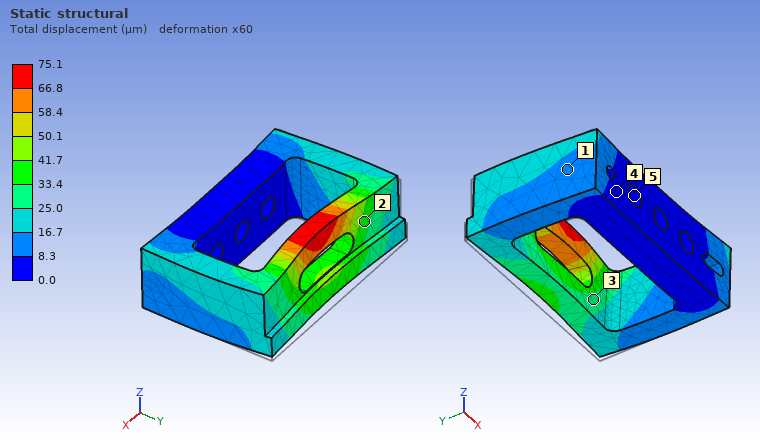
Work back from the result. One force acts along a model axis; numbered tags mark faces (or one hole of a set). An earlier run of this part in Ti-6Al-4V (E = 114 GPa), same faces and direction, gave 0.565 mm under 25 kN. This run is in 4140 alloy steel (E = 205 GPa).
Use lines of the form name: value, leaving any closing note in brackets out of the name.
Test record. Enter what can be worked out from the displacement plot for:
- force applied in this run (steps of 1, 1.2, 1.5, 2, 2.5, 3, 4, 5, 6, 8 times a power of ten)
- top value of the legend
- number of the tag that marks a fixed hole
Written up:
force applied in this run: 6 kN
top value of the legend: 75.1 µm
number of the tag that marks a fixed hole: 5
